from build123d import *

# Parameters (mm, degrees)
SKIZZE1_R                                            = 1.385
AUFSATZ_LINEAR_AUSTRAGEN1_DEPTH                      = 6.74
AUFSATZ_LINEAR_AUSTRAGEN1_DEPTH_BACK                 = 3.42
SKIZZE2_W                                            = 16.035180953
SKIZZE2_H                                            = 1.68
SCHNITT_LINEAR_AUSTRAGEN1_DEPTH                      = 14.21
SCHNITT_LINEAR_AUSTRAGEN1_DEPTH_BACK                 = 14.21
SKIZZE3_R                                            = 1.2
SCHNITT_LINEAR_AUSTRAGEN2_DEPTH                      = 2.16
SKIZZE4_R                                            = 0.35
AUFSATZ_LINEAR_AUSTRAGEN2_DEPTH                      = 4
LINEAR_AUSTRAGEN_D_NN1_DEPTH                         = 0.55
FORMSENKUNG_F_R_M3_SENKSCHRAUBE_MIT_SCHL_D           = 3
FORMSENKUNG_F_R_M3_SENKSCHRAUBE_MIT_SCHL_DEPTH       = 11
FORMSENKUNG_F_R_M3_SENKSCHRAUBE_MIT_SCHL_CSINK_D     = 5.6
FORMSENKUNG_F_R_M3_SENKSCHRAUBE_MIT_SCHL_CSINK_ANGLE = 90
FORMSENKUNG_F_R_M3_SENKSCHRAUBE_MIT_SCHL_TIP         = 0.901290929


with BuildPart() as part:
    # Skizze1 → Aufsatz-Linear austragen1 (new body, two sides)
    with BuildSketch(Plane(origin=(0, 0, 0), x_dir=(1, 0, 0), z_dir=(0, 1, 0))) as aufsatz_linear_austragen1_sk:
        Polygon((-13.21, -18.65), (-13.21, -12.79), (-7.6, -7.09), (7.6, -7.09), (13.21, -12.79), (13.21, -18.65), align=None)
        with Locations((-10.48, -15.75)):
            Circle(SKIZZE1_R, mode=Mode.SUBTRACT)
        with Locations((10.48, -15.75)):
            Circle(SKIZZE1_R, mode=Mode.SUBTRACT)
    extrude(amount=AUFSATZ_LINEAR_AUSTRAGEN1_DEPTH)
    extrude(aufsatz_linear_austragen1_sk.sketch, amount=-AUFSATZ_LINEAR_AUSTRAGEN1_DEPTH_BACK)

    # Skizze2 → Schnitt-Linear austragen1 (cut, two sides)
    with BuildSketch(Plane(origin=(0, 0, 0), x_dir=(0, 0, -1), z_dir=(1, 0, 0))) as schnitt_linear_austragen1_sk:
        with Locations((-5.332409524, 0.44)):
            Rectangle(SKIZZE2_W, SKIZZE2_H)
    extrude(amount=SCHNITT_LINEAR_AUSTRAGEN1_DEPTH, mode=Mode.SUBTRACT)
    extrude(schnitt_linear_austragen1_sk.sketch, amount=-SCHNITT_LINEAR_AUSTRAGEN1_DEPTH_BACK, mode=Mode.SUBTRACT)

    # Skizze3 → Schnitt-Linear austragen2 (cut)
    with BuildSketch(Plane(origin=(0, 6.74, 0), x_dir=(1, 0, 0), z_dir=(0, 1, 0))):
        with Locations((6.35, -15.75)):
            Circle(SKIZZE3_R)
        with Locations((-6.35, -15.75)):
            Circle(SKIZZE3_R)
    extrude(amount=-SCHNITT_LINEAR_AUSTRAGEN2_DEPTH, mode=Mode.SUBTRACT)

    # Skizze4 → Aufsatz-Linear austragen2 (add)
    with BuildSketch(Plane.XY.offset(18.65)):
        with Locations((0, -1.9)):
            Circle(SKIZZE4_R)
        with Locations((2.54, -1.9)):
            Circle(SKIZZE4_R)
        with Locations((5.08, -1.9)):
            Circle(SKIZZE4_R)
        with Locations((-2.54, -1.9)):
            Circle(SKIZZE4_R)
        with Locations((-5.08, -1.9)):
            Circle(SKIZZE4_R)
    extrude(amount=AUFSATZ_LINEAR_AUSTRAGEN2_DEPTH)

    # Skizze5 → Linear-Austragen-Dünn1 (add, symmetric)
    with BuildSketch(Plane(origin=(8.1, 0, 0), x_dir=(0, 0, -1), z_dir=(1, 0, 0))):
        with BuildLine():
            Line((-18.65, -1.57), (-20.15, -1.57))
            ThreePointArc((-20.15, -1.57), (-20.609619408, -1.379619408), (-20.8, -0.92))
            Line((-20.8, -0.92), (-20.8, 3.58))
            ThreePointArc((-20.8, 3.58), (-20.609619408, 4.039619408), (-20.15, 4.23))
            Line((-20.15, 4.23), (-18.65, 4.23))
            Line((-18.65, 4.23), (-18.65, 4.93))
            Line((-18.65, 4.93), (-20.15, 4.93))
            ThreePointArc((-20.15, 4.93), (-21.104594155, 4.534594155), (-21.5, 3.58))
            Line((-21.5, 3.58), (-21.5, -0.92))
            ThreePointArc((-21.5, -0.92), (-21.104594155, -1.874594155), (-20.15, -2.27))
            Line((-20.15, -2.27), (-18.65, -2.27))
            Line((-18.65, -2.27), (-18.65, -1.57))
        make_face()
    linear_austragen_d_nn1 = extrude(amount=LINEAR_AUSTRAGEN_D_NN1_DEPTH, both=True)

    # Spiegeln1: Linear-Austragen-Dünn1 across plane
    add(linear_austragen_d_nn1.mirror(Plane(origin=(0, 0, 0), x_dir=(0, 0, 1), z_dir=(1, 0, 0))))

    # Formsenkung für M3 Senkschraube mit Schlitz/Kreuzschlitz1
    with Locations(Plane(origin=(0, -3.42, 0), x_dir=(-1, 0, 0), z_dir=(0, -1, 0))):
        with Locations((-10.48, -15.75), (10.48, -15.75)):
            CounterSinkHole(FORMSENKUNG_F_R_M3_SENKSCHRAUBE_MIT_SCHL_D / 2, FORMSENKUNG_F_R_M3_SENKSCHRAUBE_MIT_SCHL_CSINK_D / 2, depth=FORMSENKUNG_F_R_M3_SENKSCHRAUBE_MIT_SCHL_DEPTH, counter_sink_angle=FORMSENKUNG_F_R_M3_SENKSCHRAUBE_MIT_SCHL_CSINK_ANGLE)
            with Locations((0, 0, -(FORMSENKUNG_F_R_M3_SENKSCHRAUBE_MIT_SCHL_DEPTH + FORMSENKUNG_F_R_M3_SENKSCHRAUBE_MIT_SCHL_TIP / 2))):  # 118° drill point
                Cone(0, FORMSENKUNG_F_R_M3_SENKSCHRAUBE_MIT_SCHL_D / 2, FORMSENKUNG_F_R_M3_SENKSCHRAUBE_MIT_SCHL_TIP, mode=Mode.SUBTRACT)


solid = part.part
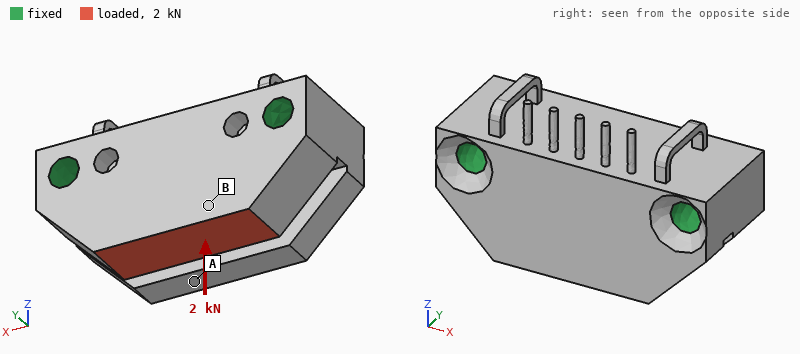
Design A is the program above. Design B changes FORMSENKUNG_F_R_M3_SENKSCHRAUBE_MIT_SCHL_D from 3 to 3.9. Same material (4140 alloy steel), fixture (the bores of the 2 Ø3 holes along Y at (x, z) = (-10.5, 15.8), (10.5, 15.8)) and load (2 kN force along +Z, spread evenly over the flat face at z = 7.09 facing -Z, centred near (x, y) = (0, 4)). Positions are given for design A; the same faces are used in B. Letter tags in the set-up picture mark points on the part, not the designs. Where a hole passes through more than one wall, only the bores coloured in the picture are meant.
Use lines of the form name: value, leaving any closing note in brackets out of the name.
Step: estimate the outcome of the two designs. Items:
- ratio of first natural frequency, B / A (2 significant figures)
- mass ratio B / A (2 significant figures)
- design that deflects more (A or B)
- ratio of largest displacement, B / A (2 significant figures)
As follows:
ratio of first natural frequency, B / A: 1.0
mass ratio B / A: 0.96
design that deflects more: A
ratio of largest displacement, B / A: 0.90
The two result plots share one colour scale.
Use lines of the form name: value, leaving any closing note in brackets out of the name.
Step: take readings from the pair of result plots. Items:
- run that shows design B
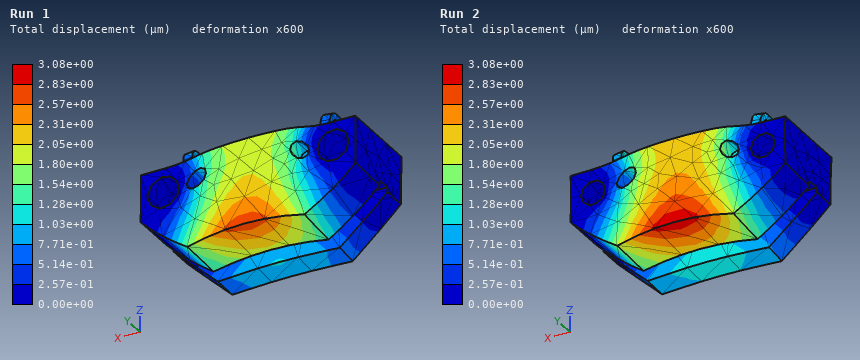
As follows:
run that shows design B: Run 1
